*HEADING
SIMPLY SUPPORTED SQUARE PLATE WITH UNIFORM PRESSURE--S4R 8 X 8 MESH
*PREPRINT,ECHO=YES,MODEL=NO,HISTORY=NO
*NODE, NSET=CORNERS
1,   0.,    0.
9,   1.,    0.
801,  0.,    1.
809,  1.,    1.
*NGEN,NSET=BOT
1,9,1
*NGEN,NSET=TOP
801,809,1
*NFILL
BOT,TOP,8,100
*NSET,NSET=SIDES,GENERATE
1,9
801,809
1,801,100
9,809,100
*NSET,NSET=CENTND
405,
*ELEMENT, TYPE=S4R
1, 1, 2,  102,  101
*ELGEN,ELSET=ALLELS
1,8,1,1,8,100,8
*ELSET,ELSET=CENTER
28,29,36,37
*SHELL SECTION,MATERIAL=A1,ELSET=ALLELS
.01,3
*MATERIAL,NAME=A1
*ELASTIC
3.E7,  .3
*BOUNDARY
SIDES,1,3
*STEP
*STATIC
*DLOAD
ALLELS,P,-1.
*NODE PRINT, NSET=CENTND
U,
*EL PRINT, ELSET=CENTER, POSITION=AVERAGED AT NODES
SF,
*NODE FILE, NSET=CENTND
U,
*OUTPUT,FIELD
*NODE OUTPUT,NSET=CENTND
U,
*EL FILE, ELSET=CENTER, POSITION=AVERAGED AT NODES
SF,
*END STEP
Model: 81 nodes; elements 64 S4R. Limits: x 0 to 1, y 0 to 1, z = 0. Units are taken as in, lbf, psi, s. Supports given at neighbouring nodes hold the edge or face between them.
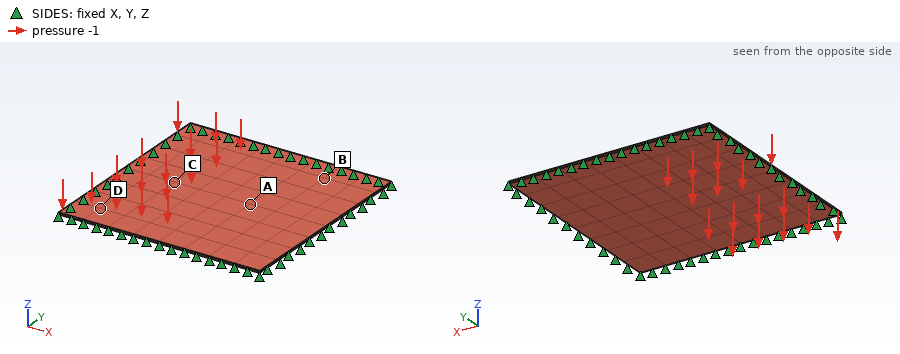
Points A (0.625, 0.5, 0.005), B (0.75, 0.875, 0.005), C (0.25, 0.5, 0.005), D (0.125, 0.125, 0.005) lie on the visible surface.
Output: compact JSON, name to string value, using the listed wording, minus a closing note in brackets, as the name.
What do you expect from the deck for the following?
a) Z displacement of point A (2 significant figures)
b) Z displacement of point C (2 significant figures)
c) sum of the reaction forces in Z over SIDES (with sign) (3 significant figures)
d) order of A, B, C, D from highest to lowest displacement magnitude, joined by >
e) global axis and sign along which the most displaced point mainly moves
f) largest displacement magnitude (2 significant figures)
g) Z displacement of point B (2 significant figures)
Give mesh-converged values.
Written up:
{"Z displacement of point A": "-0.0014 in", "Z displacement of point C": "-0.0011 in", "sum of the reaction forces in Z over SIDES (with sign)": "1.00 lbf", "order of A, B, C, D from highest to lowest displacement magnitude, joined by >": "A > C > B > D", "global axis and sign along which the most displaced point mainly moves": "-Z", "largest displacement magnitude": "0.0015 in", "Z displacement of point B": "-4.3e-04 in"}
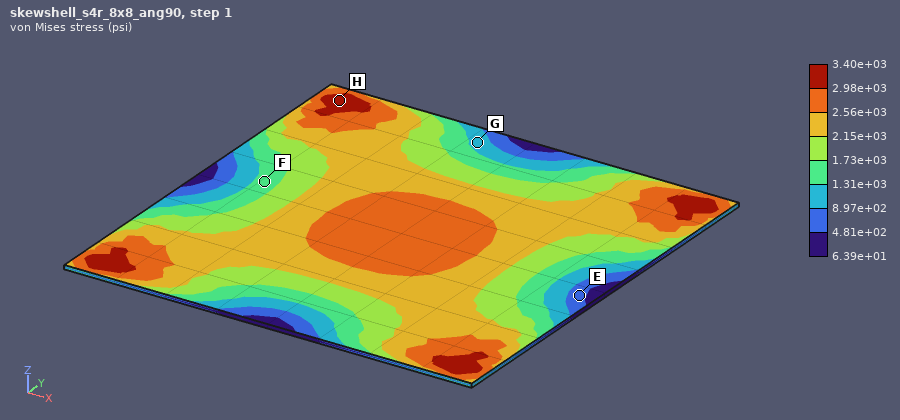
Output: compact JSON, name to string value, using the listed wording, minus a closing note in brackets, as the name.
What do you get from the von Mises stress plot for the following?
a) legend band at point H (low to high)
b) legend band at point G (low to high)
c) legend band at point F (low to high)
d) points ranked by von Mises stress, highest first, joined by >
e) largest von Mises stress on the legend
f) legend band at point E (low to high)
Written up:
{"legend band at point H": "2.98e+03 to 3.40e+03 psi", "legend band at point G": "8.97e+02 to 1.31e+03 psi", "legend band at point F": "1.31e+03 to 1.73e+03 psi", "points ranked by von Mises stress, highest first, joined by >": "H > F > G > E", "largest von Mises stress on the legend": "3.40e+03 psi", "legend band at point E": "4.81e+02 to 8.97e+02 psi"}
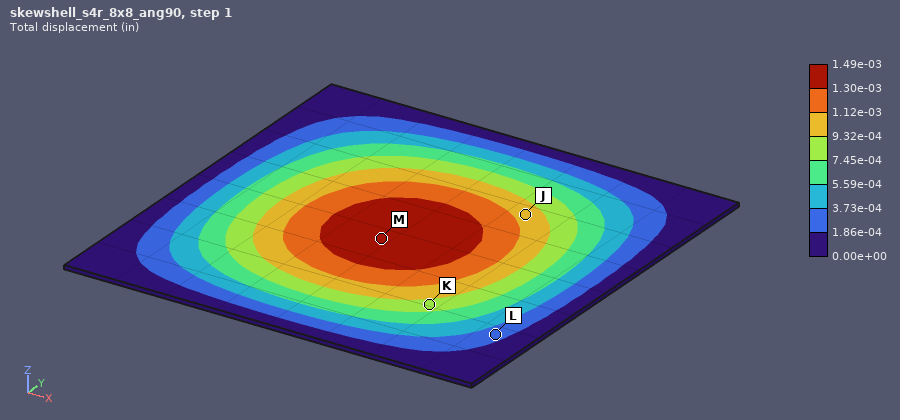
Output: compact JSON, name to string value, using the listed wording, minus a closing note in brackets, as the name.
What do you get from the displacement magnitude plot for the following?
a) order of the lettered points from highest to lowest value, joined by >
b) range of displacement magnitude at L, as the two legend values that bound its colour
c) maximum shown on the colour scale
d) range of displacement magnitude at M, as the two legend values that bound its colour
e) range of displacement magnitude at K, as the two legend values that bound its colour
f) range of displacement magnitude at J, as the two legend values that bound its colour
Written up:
{"order of the lettered points from highest to lowest value, joined by >": "M > J > K > L", "range of displacement magnitude at L, as the two legend values that bound its colour": "1.86e-04 to 3.73e-04 in", "maximum shown on the colour scale": "1.49e-03 in", "range of displacement magnitude at M, as the two legend values that bound its colour": "1.30e-03 to 1.49e-03 in", "range of displacement magnitude at K, as the two legend values that bound its colour": "7.45e-04 to 9.32e-04 in", "range of displacement magnitude at J, as the two legend values that bound its colour": "9.32e-04 to 1.12e-03 in"}
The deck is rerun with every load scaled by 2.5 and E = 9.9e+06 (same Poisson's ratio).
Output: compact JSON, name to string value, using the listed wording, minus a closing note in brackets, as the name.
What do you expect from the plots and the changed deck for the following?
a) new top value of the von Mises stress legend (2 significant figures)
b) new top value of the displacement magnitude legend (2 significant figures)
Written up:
{"new top value of the von Mises stress legend": "8500 psi", "new top value of the displacement magnitude legend": "0.011 in"}
